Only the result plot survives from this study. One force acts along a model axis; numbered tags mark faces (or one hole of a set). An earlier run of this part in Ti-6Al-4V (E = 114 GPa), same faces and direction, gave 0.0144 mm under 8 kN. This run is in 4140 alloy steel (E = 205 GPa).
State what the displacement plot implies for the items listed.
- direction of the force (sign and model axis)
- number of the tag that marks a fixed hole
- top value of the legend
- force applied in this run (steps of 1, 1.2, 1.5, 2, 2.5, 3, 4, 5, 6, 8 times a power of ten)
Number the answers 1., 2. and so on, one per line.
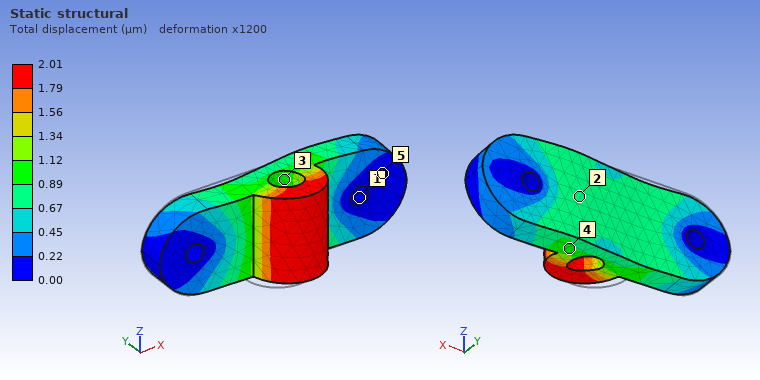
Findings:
1. +X
2. 1
3. 2.01 µm
4. 2 kN
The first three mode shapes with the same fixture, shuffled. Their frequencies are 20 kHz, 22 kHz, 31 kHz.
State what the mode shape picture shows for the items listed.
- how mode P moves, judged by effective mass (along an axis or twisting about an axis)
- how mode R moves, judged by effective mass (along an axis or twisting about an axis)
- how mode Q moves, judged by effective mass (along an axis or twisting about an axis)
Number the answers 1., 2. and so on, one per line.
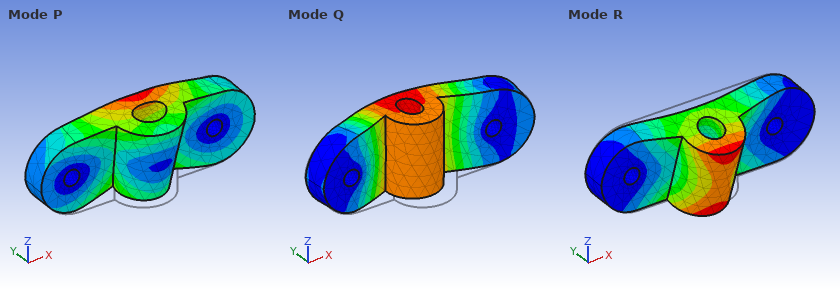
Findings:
1. along Z
2. along Z
3. along Y
